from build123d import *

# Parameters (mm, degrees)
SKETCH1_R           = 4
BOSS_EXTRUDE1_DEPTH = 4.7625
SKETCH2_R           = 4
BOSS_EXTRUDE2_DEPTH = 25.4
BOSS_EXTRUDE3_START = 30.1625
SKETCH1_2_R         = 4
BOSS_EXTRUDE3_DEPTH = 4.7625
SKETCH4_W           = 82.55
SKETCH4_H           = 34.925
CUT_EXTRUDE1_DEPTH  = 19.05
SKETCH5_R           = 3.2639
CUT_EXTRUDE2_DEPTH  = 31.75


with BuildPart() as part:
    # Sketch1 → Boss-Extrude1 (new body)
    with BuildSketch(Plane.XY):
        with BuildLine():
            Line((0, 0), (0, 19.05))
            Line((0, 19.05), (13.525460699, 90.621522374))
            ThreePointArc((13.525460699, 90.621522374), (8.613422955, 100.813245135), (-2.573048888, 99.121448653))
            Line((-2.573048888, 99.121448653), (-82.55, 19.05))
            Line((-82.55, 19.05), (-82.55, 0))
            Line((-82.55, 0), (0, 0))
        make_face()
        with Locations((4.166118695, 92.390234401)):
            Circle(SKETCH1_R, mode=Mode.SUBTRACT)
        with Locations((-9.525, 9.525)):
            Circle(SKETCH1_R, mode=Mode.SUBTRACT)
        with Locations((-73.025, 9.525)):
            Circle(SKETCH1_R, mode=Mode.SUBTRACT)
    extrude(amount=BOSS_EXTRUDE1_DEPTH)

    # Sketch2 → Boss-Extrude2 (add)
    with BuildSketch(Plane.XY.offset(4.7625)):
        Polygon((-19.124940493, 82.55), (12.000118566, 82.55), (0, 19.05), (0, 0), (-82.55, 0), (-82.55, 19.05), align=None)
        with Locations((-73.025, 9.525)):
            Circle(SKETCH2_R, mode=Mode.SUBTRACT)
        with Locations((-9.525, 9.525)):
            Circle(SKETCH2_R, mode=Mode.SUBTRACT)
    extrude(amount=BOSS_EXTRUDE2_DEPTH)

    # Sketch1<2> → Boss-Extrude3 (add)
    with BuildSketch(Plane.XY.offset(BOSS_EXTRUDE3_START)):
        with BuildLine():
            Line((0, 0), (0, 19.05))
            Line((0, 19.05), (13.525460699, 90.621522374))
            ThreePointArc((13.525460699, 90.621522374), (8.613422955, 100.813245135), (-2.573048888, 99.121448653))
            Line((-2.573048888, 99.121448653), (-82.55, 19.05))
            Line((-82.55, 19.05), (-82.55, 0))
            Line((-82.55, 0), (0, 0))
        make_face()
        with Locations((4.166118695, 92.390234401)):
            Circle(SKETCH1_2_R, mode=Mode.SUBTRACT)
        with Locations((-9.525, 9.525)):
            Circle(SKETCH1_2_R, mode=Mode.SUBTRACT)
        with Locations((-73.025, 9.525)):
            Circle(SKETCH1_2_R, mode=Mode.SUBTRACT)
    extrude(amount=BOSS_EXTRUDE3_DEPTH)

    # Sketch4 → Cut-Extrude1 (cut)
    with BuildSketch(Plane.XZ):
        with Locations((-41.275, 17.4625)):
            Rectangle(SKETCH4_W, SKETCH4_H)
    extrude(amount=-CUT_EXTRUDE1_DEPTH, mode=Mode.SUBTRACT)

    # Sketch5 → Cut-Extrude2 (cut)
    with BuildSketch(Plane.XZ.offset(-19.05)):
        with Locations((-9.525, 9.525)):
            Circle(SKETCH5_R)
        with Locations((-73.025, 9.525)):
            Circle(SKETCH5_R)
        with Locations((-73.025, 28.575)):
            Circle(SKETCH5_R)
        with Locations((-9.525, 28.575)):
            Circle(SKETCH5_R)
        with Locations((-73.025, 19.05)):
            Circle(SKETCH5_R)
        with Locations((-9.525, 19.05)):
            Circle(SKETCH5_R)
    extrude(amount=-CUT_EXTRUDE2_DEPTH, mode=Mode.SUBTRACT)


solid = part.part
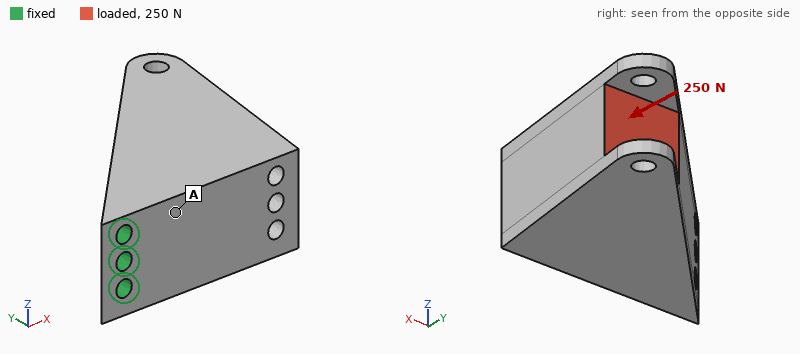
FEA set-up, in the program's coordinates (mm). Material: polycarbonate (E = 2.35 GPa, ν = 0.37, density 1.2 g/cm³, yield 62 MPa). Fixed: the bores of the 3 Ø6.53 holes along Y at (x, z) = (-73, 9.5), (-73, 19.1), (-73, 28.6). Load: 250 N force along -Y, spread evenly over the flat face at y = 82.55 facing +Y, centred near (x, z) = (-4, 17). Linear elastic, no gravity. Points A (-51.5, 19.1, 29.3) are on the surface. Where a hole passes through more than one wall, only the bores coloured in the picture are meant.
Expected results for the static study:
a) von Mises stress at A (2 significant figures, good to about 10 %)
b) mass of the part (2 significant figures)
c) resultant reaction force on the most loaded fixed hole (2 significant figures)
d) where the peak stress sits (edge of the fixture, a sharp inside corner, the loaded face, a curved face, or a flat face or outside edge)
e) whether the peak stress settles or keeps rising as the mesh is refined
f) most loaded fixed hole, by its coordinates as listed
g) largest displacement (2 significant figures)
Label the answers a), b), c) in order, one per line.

a) 3.7 MPa
b) 150 g
c) 130 N
d) edge of the fixture
e) keeps rising
f) (-73, 19.1)
g) 1.2 mm
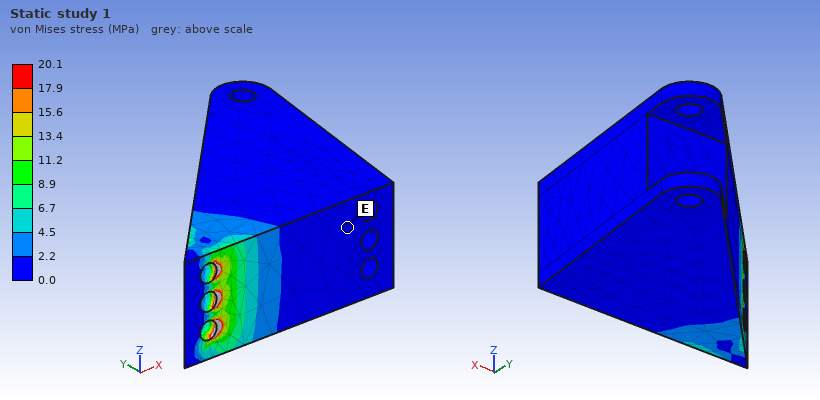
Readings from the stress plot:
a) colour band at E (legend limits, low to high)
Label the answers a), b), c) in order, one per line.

a) 0.0 to 2.2 MPa
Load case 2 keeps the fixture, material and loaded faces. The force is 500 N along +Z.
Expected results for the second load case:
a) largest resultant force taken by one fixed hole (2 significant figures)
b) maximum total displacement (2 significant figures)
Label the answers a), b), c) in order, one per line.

a) 1.8 kN
b) 1.3 mm
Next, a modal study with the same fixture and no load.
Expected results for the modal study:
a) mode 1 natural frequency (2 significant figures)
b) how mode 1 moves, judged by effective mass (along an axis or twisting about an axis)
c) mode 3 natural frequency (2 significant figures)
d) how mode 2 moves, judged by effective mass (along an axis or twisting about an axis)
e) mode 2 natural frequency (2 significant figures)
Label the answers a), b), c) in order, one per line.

a) 280 Hz
b) along Y
c) 1100 Hz
d) along Z
e) 510 Hz
